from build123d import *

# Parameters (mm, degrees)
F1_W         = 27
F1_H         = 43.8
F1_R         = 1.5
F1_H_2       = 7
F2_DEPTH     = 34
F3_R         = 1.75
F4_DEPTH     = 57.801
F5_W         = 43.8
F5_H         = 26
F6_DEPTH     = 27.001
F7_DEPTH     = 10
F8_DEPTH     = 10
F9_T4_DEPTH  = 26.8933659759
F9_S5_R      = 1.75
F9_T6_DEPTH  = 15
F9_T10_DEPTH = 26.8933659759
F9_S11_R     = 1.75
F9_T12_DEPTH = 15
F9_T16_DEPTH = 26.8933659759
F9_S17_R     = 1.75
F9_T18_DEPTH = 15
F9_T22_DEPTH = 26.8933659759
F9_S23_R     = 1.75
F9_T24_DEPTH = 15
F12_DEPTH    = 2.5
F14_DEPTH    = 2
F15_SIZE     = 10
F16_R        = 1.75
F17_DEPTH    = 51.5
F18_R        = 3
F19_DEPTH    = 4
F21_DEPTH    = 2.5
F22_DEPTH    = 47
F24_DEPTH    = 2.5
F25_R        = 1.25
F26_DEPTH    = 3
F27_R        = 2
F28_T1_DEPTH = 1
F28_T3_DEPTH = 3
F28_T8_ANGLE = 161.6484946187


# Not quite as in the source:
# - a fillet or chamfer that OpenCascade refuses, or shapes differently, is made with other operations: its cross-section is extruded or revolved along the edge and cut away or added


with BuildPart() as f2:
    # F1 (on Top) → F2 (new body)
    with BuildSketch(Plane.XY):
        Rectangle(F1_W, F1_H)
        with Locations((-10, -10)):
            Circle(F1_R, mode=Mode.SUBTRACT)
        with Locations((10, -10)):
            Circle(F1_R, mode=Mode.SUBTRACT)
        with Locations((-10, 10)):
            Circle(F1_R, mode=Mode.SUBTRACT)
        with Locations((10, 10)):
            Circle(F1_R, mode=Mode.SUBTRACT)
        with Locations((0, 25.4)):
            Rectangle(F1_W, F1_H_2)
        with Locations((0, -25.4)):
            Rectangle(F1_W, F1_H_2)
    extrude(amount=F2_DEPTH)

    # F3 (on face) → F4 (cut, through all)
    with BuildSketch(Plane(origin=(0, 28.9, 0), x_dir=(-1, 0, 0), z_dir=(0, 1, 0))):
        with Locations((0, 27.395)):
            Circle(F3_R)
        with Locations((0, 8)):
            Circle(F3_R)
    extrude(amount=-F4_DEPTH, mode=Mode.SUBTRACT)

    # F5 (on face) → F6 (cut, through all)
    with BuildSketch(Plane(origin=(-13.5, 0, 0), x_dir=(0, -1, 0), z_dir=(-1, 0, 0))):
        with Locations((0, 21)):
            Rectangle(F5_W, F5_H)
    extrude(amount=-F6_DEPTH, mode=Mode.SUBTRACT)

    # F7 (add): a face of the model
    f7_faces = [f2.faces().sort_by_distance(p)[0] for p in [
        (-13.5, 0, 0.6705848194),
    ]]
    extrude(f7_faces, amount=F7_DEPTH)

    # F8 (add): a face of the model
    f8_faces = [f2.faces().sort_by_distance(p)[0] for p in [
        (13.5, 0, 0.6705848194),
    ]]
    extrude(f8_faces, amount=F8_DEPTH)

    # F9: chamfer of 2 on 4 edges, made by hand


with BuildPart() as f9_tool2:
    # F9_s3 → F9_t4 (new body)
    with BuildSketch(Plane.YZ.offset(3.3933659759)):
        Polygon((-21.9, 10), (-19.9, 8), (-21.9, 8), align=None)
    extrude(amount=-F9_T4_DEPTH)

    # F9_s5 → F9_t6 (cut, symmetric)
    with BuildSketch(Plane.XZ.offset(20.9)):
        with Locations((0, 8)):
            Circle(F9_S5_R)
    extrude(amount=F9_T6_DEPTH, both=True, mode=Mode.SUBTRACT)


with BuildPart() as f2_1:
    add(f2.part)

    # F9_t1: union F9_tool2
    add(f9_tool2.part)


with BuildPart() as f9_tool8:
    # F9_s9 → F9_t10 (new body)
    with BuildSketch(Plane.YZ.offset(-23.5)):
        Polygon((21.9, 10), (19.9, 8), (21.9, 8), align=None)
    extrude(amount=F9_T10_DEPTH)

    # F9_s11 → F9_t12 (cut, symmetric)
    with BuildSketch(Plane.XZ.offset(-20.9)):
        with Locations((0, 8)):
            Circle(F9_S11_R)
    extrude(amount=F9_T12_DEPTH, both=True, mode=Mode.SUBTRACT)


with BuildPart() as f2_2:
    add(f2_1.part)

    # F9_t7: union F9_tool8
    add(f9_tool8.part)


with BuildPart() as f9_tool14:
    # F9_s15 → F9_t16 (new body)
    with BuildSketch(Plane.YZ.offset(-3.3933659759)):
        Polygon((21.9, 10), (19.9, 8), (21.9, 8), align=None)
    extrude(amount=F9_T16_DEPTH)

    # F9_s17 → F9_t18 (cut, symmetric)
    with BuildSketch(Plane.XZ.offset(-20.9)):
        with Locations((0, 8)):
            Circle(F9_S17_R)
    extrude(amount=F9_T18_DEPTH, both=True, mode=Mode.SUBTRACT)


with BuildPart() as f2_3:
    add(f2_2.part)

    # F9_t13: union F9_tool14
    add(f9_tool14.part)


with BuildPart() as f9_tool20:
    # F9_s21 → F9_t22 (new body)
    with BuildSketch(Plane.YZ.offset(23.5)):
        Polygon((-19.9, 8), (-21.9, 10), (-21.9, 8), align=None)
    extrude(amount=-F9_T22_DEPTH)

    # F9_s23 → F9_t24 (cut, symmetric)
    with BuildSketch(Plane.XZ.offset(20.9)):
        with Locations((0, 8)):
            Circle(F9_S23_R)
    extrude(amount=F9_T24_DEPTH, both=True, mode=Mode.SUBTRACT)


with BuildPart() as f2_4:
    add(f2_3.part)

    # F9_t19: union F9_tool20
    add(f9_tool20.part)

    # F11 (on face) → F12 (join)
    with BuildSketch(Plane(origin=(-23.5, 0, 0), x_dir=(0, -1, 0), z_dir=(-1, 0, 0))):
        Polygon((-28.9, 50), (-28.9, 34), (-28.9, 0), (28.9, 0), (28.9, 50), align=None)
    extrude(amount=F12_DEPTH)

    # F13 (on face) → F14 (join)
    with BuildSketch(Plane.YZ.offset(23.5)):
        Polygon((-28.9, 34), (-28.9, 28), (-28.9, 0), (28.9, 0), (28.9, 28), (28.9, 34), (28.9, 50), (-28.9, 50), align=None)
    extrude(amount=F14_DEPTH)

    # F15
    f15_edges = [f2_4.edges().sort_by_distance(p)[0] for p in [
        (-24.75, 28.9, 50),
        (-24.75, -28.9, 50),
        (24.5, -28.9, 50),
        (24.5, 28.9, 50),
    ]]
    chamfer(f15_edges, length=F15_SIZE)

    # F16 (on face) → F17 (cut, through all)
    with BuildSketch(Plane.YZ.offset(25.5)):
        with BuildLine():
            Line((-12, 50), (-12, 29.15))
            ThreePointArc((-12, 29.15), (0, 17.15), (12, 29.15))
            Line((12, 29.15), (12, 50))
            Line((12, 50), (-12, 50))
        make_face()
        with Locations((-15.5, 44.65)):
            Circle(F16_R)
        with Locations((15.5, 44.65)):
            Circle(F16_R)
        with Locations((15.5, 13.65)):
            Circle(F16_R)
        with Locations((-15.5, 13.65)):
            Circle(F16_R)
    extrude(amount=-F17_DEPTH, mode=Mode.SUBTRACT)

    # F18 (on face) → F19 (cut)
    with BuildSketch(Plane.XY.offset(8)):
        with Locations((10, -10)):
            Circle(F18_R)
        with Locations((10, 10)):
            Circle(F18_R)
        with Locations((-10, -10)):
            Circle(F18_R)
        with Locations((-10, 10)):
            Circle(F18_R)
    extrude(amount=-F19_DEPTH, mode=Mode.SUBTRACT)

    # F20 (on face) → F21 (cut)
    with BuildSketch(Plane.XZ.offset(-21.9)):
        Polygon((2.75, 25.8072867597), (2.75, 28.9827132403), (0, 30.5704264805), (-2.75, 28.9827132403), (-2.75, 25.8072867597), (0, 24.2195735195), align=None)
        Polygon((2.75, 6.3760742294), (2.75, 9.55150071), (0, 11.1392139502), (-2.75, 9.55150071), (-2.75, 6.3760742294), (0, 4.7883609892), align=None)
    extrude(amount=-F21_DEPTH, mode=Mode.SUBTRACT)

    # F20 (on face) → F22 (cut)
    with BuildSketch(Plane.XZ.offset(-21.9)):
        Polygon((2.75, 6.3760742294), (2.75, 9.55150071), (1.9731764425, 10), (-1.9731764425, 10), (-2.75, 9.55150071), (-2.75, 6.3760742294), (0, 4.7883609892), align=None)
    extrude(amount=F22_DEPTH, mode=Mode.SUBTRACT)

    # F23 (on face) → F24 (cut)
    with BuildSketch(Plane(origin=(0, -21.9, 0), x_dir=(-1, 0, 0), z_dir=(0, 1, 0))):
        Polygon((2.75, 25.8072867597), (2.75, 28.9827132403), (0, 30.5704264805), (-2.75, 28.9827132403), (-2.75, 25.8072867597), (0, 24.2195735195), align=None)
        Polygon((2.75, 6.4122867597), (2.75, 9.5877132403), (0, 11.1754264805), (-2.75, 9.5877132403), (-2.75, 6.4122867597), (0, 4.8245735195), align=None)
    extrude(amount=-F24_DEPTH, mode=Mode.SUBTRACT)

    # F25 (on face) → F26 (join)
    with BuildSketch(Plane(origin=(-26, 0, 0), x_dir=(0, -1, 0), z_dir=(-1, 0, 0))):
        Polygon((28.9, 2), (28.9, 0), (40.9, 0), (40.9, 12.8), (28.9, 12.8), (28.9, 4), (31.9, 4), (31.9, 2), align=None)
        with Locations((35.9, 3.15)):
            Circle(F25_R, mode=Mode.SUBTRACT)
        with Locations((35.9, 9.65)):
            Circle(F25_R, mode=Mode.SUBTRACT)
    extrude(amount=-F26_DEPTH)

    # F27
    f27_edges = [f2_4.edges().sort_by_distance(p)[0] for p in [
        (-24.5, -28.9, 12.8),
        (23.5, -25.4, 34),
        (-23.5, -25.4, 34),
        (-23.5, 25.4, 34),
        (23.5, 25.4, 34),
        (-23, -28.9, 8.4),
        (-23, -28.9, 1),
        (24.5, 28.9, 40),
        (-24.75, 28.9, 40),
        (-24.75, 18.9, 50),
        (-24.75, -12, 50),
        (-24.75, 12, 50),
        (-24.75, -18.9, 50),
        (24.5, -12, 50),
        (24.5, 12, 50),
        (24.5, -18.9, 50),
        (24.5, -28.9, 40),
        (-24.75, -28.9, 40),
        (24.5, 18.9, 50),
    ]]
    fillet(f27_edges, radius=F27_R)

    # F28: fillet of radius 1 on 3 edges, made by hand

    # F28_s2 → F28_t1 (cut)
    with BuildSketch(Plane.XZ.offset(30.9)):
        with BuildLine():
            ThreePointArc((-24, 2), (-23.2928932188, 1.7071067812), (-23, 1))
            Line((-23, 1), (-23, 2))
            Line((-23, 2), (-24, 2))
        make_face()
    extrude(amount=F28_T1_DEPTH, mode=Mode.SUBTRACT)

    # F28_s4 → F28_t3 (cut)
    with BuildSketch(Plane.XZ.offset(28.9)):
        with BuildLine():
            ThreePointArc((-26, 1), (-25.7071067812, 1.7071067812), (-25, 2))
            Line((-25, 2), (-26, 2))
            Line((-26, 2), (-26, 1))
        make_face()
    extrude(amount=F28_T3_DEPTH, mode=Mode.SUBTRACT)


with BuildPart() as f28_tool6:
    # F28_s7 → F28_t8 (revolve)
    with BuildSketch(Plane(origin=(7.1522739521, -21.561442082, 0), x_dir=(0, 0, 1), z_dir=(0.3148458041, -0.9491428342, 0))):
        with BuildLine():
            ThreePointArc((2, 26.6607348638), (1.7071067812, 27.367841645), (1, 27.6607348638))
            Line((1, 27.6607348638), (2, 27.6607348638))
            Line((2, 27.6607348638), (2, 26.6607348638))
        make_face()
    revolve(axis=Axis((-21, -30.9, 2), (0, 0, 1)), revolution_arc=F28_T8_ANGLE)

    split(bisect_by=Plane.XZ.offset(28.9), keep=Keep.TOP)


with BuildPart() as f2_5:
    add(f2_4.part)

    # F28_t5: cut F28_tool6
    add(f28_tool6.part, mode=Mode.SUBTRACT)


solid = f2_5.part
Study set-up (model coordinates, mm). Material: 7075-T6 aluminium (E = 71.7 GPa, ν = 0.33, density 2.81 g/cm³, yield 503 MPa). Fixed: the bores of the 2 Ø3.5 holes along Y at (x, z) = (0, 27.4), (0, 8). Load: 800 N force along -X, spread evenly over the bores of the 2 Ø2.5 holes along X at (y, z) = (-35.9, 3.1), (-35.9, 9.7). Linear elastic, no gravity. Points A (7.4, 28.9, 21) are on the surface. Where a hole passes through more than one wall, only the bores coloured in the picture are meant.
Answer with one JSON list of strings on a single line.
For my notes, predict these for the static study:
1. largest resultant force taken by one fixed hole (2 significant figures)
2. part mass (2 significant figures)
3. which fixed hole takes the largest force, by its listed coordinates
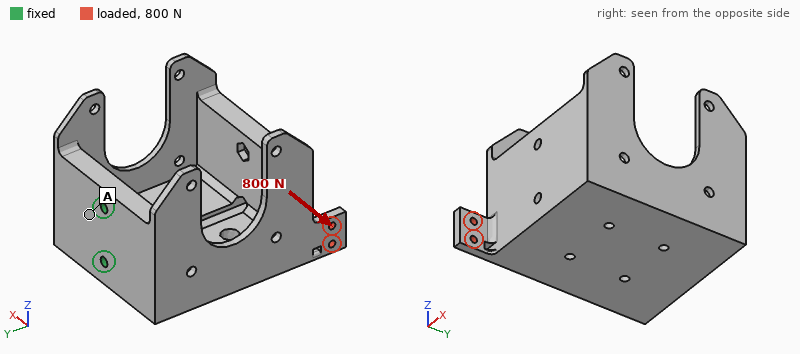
["770 N", "130 g", "(0, 8)"]
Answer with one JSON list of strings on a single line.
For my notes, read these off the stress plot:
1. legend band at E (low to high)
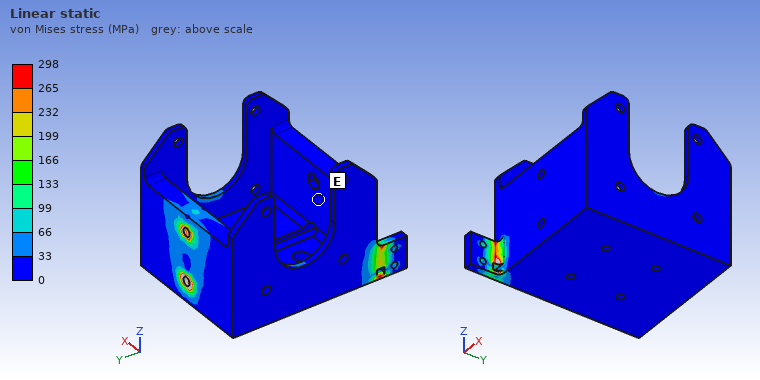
["0 to 33 MPa"]
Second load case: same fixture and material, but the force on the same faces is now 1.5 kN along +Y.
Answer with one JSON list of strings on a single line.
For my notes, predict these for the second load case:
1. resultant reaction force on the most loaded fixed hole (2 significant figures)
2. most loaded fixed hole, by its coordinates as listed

["1.5 kN", "(0, 8)"]
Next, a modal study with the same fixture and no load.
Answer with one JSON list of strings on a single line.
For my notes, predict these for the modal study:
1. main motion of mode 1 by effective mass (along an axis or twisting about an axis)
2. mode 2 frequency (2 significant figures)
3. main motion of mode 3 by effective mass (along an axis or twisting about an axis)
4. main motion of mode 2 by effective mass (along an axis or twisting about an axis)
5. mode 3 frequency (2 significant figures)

["along X", "1300 Hz", "twisting about Y", "along Z", "2600 Hz"]
